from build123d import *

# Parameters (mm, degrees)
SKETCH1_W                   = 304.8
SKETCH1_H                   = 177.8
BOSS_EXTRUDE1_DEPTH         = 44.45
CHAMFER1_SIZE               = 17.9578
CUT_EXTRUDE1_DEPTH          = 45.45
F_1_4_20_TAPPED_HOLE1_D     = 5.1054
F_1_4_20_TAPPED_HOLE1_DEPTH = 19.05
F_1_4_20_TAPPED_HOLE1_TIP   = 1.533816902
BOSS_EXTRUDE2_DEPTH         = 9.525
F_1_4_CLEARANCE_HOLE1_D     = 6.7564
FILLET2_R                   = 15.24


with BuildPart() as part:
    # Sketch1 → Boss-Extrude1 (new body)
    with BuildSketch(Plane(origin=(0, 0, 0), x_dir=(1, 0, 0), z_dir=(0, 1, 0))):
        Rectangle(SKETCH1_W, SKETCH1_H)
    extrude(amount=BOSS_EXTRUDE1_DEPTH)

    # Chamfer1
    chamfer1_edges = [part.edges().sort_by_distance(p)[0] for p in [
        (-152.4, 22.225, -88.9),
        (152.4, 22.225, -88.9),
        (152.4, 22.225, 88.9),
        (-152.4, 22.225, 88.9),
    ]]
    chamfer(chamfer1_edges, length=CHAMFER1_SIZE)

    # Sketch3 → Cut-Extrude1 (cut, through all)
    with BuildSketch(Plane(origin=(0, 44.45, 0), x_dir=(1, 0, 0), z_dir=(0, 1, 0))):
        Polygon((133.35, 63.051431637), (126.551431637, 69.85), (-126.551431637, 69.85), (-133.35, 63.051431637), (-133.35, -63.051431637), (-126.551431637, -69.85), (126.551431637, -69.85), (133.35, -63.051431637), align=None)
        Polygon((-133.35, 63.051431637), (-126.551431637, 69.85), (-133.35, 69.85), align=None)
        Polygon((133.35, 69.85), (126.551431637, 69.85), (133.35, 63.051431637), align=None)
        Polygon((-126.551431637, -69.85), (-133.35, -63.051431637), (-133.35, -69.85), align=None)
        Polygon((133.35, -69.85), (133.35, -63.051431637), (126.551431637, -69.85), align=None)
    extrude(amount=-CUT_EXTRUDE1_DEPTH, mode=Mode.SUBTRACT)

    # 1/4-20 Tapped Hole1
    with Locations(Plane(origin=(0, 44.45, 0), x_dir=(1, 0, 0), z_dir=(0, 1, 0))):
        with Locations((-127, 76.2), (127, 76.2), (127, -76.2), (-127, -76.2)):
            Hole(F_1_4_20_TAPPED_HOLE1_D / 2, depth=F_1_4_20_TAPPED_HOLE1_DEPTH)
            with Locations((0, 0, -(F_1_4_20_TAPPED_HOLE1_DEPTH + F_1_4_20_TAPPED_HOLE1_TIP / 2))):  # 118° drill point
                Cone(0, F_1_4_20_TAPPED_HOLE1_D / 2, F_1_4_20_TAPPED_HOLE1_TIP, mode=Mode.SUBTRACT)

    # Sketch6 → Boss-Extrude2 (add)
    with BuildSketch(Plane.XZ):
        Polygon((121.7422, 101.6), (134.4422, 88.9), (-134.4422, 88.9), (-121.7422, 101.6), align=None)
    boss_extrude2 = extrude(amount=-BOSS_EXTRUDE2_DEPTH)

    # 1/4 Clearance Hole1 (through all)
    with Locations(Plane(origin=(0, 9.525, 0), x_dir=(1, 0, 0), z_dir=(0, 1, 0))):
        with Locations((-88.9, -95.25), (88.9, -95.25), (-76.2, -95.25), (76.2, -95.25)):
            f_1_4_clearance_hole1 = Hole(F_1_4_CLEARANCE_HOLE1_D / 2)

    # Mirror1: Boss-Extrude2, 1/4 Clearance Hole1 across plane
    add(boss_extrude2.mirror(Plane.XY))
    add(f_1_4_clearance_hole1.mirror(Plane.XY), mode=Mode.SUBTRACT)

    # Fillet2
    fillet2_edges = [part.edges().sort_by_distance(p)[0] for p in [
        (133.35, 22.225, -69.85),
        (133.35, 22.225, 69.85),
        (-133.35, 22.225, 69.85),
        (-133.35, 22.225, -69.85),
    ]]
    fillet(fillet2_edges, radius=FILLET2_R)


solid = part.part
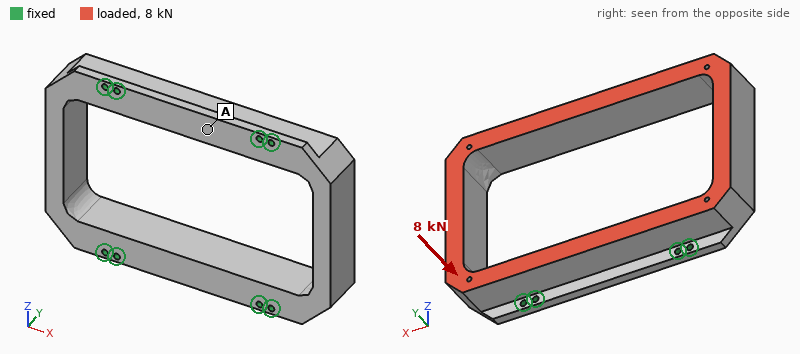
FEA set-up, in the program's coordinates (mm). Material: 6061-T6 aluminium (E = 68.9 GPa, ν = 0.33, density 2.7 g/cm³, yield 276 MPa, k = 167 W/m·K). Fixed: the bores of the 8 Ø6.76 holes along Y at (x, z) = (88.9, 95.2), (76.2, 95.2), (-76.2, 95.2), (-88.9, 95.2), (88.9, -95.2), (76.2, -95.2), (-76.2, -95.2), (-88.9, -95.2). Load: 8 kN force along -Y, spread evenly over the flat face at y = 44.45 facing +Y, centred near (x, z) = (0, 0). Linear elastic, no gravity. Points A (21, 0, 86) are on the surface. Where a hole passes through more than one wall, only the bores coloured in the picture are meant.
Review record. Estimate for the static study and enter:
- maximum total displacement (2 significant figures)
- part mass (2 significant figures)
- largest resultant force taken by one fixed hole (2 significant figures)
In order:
36 µm
2.1 kg
1.6 kN
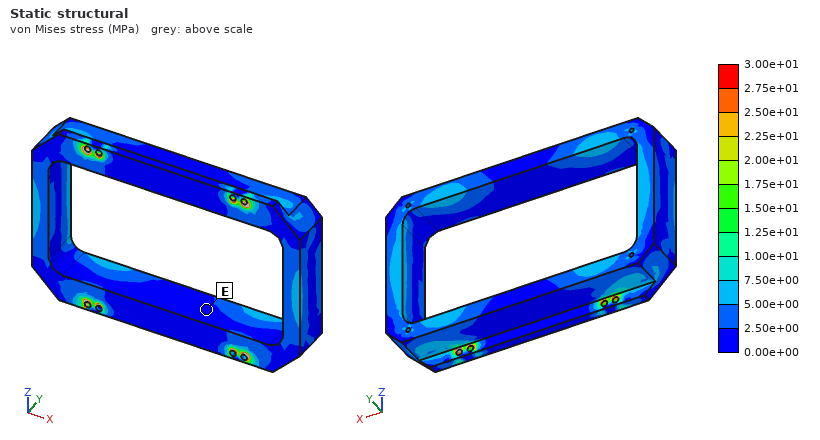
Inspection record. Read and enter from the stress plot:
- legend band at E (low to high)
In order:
0.00e+00 to 2.50e+00 MPa
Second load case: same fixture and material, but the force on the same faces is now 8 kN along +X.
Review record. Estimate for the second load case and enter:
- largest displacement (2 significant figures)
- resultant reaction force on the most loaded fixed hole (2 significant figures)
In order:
41 µm
1.4 kN
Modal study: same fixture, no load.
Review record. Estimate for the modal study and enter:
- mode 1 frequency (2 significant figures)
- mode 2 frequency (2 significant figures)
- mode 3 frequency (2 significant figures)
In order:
1800 Hz
1900 Hz
2300 Hz
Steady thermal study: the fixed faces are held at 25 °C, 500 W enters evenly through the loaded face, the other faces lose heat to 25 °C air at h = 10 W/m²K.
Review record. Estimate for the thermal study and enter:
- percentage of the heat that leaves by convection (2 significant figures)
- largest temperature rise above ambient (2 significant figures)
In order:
6.3 %
49 K
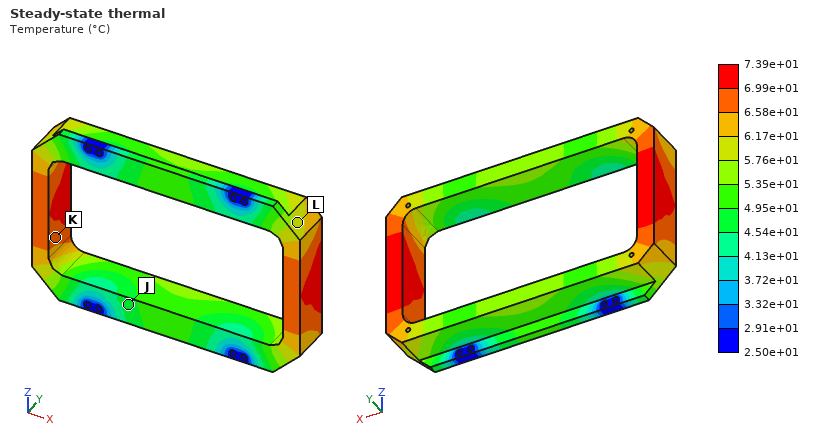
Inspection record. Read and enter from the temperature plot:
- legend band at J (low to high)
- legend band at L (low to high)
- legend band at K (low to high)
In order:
4.54e+01 to 4.95e+01 °C
5.76e+01 to 6.17e+01 °C
6.58e+01 to 6.99e+01 °C
